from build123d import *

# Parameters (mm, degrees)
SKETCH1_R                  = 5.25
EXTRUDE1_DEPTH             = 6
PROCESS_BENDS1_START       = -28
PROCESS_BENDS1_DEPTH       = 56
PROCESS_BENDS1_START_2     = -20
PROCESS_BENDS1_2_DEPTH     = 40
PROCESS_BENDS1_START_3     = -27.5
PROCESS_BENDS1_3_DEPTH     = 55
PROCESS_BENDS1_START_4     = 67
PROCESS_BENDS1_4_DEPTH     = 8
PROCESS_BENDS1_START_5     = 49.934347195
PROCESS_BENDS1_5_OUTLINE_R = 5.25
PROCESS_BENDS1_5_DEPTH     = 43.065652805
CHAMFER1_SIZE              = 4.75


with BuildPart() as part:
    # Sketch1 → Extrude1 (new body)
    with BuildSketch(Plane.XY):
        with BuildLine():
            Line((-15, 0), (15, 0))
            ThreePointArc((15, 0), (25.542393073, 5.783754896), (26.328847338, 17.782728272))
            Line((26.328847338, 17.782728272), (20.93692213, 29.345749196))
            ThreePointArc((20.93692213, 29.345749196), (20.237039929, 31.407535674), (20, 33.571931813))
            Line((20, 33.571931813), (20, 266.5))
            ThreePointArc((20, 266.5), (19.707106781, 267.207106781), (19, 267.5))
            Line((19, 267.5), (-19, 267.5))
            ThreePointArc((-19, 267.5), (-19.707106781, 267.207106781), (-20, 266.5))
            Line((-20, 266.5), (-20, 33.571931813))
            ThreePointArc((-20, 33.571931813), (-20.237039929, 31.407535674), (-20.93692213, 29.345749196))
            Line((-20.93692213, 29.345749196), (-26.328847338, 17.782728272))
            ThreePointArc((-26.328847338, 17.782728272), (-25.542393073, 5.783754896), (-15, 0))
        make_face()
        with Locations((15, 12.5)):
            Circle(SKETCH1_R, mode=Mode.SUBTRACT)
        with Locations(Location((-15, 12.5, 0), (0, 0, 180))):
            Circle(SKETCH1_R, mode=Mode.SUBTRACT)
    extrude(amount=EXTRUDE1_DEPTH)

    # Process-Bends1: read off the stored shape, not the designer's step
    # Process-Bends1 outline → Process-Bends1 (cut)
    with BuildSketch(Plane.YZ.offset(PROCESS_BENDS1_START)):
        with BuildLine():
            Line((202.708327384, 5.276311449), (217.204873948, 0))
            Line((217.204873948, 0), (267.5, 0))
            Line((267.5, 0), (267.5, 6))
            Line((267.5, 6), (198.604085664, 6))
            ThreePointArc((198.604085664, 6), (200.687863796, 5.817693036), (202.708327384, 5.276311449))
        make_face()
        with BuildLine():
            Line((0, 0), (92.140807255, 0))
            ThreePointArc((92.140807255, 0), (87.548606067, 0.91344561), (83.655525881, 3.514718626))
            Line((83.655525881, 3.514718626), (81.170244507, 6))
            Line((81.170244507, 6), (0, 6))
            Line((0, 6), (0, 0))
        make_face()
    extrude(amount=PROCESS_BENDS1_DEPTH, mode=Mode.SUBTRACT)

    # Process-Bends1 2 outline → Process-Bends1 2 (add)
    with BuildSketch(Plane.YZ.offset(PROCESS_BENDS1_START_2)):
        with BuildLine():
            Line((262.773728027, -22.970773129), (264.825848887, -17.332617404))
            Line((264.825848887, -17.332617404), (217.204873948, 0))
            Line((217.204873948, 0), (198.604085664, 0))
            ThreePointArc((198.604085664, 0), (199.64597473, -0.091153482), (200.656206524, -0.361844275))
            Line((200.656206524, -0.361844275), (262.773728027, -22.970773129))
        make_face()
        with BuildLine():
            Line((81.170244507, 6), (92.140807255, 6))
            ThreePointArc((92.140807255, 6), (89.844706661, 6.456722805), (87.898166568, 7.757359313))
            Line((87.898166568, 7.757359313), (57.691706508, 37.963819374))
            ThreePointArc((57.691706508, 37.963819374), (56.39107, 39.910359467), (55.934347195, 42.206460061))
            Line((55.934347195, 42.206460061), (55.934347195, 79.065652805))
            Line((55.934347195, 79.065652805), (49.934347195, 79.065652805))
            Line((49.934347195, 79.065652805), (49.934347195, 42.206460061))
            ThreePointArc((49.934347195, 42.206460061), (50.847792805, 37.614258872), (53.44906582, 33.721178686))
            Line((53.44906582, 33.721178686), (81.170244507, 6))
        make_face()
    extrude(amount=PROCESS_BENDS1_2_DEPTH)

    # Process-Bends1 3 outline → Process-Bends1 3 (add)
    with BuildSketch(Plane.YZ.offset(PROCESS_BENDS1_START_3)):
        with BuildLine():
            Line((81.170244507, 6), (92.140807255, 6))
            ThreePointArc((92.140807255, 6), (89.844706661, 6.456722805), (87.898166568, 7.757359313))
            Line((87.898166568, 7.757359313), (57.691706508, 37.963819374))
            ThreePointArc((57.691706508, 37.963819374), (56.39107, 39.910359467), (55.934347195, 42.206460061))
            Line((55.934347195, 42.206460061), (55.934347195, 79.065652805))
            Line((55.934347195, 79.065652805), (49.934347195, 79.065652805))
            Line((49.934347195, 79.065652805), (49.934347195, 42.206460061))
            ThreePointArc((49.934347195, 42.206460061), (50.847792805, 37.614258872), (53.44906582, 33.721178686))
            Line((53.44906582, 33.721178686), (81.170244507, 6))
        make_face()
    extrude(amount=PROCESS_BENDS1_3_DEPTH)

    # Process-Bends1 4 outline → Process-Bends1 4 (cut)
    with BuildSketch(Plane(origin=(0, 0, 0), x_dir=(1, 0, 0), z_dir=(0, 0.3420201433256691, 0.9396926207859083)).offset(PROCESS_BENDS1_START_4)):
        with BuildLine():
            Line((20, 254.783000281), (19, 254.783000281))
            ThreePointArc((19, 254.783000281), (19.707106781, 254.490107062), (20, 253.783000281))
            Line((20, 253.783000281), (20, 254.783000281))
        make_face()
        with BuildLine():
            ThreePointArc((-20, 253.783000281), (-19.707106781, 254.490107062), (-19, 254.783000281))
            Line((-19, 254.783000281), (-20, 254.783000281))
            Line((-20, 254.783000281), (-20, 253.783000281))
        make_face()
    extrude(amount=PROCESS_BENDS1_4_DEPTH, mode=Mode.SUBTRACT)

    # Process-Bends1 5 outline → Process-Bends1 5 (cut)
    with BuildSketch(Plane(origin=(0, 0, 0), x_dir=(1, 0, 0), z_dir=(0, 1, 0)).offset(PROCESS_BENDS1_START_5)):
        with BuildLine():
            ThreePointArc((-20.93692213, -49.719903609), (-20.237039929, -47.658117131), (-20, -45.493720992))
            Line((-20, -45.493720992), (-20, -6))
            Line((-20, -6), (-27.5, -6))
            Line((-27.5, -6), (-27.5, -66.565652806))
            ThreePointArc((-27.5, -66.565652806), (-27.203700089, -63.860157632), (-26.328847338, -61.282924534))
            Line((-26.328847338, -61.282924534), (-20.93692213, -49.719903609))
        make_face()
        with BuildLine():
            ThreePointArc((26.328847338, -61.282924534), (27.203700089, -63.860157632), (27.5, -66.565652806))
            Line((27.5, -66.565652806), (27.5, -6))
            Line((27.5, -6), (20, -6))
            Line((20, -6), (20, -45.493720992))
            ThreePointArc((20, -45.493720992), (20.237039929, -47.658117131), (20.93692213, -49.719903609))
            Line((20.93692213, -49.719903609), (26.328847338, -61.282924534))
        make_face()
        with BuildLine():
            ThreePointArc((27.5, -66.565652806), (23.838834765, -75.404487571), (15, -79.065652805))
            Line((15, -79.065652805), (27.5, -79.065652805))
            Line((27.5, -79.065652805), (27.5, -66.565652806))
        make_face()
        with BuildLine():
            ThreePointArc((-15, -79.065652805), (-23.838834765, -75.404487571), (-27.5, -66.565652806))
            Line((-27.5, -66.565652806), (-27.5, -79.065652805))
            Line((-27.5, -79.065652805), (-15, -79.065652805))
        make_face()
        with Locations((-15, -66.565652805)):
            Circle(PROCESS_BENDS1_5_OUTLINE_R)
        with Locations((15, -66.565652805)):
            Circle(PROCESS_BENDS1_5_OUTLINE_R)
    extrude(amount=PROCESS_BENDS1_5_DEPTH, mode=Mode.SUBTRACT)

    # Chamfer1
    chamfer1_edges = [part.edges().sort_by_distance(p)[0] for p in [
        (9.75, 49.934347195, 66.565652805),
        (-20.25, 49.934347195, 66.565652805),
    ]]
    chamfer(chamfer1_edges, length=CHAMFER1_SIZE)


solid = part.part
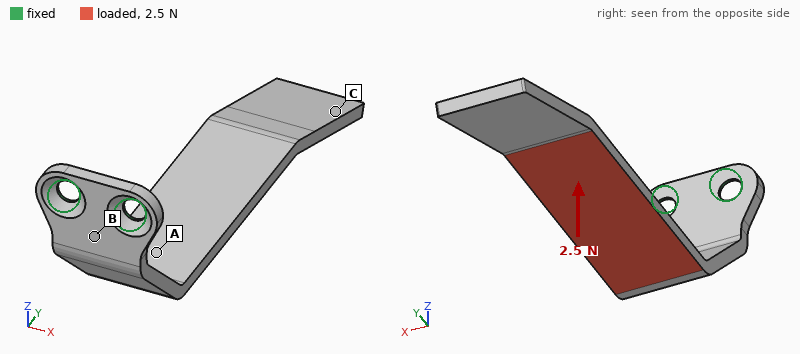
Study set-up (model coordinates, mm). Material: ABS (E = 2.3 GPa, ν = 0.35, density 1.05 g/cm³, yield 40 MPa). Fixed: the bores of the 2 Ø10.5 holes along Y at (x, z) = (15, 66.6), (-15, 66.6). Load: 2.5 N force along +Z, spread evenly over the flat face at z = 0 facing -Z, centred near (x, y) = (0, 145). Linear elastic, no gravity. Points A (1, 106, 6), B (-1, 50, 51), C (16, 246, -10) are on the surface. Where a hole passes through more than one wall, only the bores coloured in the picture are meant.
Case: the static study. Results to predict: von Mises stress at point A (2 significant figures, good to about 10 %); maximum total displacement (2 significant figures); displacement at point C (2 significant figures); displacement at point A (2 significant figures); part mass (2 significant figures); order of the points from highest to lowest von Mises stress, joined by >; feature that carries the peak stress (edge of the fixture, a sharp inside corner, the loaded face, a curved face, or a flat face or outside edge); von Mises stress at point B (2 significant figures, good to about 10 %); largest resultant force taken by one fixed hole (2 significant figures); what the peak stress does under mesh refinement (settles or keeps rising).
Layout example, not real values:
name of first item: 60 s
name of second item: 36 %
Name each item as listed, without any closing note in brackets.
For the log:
von Mises stress at point A: 0.42 MPa
maximum total displacement: 2.6 mm
displacement at point C: 2.3 mm
displacement at point A: 0.57 mm
part mass: 68 g
order of the points from highest to lowest von Mises stress, joined by >: B > A > C
feature that carries the peak stress: edge of the fixture
von Mises stress at point B: 0.91 MPa
largest resultant force taken by one fixed hole: 4.3 N
what the peak stress does under mesh refinement: keeps rising
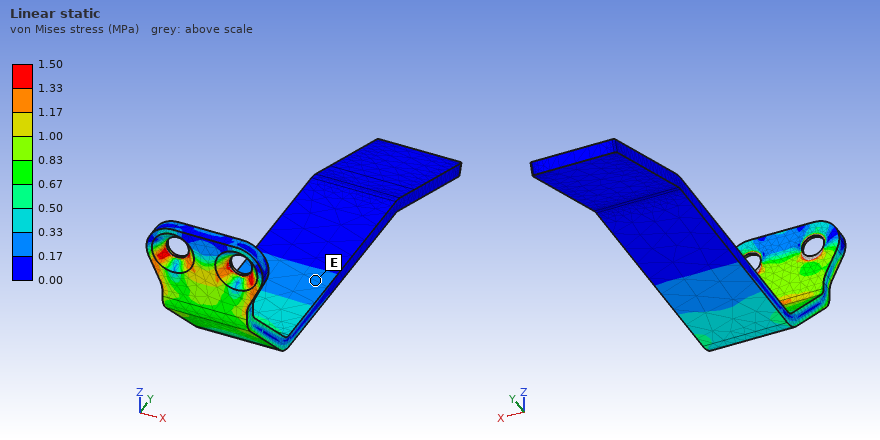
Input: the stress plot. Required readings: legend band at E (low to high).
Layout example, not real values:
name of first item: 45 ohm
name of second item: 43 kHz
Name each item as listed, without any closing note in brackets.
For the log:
legend band at E: 0.17 to 0.33 MPa
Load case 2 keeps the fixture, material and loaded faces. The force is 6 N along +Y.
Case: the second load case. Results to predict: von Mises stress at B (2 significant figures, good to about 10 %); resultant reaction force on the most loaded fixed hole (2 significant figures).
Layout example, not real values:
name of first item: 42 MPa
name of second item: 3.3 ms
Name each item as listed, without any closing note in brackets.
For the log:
von Mises stress at B: 1.3 MPa
resultant reaction force on the most loaded fixed hole: 6.9 N
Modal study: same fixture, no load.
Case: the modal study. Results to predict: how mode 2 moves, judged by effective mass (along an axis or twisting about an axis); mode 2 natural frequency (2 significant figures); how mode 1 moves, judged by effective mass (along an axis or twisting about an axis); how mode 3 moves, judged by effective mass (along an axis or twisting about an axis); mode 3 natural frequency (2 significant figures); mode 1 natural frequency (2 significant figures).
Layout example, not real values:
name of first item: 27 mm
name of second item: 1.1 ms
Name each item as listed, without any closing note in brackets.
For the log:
how mode 2 moves, judged by effective mass: along X
mode 2 natural frequency: 45 Hz
how mode 1 moves, judged by effective mass: along Z
how mode 3 moves, judged by effective mass: along Y
mode 3 natural frequency: 120 Hz
mode 1 natural frequency: 22 Hz
